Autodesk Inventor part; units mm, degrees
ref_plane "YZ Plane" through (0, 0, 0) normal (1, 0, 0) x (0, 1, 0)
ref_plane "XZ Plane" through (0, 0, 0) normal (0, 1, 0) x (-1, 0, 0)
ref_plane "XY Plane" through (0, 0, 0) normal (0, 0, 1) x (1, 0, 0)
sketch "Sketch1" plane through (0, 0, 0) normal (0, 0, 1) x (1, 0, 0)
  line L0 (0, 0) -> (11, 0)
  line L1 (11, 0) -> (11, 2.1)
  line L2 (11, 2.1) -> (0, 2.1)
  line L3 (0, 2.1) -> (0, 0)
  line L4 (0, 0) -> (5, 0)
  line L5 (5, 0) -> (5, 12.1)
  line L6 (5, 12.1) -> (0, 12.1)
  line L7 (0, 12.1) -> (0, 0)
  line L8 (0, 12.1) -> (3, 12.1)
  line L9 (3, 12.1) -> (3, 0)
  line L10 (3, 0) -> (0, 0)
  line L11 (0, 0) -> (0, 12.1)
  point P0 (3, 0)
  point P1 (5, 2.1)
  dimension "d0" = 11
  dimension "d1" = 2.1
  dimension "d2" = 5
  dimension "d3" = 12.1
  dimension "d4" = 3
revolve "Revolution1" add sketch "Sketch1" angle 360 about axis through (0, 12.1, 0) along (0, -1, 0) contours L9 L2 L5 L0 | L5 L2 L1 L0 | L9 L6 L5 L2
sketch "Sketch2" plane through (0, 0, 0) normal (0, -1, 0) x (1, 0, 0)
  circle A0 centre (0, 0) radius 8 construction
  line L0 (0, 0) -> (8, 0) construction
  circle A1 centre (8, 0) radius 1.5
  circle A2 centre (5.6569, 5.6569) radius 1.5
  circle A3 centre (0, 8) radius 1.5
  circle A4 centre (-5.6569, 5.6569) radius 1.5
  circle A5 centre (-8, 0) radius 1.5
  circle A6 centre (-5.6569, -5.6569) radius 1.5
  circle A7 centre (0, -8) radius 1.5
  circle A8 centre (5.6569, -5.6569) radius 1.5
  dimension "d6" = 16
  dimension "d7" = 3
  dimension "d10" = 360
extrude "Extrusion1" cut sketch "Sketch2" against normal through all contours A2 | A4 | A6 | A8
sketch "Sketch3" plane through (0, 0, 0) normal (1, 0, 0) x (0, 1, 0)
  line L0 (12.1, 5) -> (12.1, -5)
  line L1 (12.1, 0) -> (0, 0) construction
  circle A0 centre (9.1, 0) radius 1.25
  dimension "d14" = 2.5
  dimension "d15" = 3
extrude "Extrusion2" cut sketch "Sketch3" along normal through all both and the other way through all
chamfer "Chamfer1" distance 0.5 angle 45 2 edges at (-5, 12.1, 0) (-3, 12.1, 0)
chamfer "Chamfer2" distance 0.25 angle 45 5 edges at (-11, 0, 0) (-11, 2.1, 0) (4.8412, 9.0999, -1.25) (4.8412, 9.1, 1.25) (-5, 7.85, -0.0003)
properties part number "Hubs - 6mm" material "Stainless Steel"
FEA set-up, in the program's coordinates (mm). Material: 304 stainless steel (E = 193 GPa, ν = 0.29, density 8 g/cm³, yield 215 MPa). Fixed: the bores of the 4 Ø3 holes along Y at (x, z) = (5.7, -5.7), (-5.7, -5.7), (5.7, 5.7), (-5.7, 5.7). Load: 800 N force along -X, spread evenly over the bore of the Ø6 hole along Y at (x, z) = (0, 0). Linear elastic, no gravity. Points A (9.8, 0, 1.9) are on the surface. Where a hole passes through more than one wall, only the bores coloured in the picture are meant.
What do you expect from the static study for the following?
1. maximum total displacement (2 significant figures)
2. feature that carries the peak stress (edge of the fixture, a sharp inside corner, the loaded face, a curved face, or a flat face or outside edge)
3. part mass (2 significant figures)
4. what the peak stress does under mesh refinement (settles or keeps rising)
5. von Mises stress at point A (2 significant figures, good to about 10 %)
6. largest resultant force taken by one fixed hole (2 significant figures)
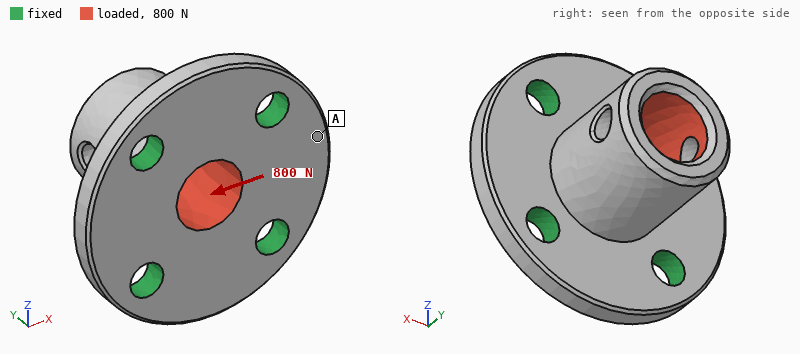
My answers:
5.5 µm
edge of the fixture
9.2 g
keeps rising
13 MPa
290 N
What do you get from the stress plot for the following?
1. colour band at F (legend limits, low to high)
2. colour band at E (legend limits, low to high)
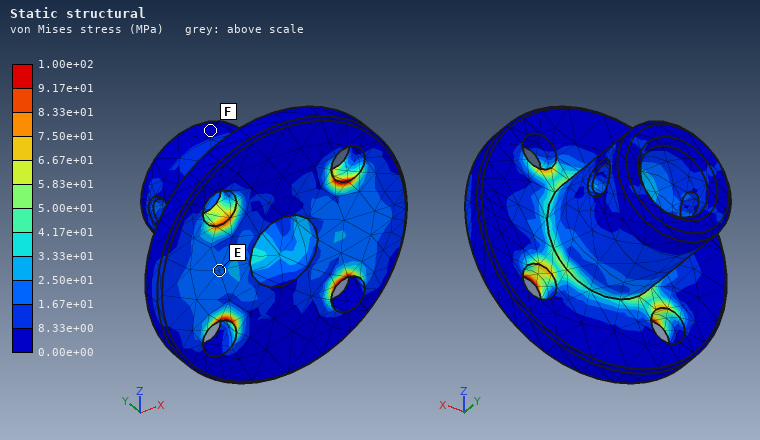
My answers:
0.00e+00 to 8.33e+00 MPa
1.67e+01 to 2.50e+01 MPa
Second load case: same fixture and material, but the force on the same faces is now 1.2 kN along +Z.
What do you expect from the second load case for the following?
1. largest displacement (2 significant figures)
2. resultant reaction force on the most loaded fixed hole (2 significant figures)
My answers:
8.7 µm
430 N
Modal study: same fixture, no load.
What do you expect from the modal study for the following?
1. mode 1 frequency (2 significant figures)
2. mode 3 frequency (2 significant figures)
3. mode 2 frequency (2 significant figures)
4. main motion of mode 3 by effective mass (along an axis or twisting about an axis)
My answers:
31 kHz
54 kHz
32 kHz
along Y
